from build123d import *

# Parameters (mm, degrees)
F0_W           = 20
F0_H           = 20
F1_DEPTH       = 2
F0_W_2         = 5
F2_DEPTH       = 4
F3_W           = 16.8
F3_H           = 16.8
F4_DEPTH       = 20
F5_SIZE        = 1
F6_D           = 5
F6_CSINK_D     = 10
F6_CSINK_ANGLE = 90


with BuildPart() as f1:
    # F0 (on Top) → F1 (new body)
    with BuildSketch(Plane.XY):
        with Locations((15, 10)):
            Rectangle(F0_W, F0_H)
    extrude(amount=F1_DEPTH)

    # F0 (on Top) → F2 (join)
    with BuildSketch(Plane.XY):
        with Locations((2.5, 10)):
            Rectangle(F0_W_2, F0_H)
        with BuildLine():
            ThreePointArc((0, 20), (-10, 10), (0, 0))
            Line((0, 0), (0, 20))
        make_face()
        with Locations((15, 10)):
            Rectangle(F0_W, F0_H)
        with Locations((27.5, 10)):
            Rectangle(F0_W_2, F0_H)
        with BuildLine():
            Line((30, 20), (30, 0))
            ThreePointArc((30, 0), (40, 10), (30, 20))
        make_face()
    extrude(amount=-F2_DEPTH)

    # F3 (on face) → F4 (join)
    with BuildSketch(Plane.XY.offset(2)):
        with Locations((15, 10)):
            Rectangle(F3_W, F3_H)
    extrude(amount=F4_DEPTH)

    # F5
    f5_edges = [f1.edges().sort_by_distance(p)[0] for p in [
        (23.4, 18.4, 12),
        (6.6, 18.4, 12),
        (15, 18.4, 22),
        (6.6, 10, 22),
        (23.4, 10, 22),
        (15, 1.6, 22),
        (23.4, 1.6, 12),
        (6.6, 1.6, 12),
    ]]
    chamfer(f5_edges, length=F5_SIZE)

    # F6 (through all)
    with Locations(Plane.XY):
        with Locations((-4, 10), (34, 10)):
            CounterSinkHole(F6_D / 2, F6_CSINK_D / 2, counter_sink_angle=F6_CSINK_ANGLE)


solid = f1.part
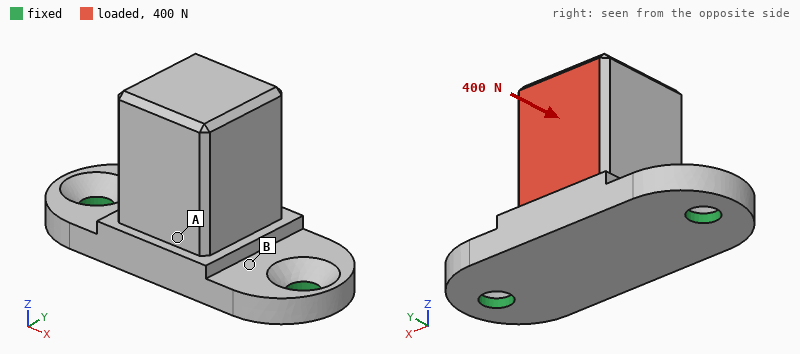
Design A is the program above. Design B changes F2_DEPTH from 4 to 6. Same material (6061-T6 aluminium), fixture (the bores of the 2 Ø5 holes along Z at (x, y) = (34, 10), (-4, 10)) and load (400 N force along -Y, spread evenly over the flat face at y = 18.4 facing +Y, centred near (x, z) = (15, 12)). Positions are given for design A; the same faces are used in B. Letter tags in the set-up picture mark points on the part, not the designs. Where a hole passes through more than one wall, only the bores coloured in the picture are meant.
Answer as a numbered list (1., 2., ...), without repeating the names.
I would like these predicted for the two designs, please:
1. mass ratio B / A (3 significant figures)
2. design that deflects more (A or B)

1. 1.18
2. A
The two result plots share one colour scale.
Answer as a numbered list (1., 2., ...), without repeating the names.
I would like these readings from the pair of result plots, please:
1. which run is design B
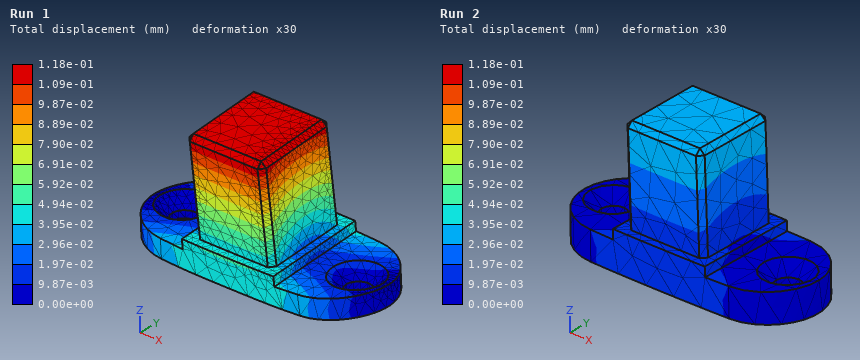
1. Run 2
